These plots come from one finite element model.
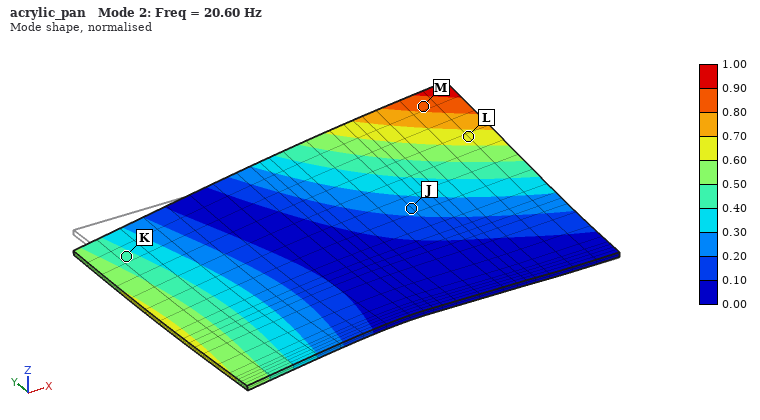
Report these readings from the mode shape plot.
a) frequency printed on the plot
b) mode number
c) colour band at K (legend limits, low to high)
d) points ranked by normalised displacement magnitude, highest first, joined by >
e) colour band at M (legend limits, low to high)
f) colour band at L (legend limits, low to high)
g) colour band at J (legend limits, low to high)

20.60 Hz
2
0.40 to 0.50
M > L > K > J
0.80 to 0.90
0.60 to 0.70
0.20 to 0.30
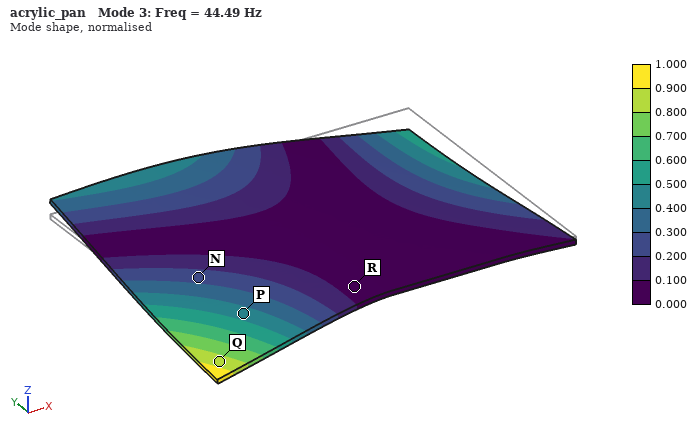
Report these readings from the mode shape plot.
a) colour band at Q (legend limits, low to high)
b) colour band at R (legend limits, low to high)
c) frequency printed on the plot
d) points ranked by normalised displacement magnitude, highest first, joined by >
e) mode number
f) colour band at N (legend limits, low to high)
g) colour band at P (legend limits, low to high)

0.800 to 0.900
0.000 to 0.100
44.49 Hz
Q > P > N > R
3
0.200 to 0.300
0.400 to 0.500
